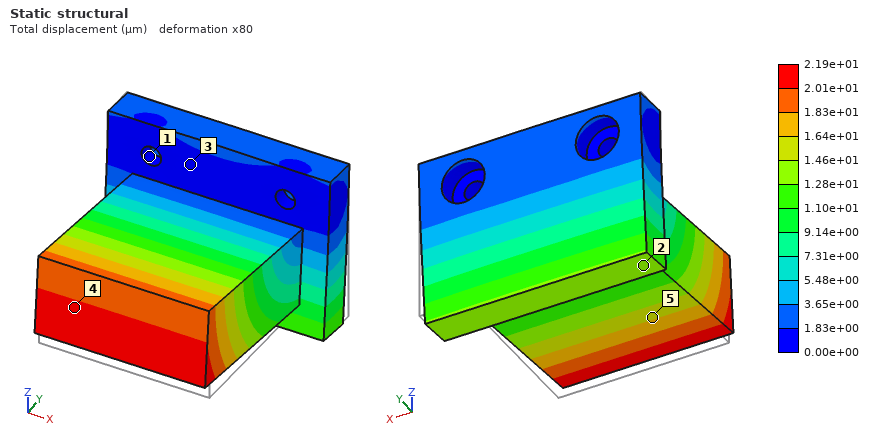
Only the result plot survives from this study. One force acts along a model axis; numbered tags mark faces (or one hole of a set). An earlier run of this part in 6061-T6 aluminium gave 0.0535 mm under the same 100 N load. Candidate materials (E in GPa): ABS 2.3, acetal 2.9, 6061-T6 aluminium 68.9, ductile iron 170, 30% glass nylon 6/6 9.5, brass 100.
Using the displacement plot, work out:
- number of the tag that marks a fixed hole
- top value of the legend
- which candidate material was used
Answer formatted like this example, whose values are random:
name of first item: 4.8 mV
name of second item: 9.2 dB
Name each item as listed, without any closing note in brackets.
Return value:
number of the tag that marks a fixed hole: 1
top value of the legend: 2.19e+01 µm
which candidate material was used: ductile iron
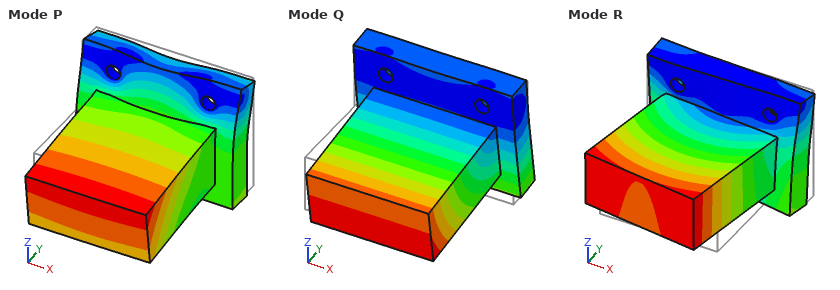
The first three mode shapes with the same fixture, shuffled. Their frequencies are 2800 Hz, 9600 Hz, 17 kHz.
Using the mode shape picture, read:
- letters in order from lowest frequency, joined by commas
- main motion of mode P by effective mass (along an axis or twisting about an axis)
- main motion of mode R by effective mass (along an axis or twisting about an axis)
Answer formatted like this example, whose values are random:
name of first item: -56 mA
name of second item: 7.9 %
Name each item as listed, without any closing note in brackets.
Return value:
letters in order from lowest frequency, joined by commas: Q, R, P
main motion of mode P by effective mass: along Y
main motion of mode R by effective mass: along X
